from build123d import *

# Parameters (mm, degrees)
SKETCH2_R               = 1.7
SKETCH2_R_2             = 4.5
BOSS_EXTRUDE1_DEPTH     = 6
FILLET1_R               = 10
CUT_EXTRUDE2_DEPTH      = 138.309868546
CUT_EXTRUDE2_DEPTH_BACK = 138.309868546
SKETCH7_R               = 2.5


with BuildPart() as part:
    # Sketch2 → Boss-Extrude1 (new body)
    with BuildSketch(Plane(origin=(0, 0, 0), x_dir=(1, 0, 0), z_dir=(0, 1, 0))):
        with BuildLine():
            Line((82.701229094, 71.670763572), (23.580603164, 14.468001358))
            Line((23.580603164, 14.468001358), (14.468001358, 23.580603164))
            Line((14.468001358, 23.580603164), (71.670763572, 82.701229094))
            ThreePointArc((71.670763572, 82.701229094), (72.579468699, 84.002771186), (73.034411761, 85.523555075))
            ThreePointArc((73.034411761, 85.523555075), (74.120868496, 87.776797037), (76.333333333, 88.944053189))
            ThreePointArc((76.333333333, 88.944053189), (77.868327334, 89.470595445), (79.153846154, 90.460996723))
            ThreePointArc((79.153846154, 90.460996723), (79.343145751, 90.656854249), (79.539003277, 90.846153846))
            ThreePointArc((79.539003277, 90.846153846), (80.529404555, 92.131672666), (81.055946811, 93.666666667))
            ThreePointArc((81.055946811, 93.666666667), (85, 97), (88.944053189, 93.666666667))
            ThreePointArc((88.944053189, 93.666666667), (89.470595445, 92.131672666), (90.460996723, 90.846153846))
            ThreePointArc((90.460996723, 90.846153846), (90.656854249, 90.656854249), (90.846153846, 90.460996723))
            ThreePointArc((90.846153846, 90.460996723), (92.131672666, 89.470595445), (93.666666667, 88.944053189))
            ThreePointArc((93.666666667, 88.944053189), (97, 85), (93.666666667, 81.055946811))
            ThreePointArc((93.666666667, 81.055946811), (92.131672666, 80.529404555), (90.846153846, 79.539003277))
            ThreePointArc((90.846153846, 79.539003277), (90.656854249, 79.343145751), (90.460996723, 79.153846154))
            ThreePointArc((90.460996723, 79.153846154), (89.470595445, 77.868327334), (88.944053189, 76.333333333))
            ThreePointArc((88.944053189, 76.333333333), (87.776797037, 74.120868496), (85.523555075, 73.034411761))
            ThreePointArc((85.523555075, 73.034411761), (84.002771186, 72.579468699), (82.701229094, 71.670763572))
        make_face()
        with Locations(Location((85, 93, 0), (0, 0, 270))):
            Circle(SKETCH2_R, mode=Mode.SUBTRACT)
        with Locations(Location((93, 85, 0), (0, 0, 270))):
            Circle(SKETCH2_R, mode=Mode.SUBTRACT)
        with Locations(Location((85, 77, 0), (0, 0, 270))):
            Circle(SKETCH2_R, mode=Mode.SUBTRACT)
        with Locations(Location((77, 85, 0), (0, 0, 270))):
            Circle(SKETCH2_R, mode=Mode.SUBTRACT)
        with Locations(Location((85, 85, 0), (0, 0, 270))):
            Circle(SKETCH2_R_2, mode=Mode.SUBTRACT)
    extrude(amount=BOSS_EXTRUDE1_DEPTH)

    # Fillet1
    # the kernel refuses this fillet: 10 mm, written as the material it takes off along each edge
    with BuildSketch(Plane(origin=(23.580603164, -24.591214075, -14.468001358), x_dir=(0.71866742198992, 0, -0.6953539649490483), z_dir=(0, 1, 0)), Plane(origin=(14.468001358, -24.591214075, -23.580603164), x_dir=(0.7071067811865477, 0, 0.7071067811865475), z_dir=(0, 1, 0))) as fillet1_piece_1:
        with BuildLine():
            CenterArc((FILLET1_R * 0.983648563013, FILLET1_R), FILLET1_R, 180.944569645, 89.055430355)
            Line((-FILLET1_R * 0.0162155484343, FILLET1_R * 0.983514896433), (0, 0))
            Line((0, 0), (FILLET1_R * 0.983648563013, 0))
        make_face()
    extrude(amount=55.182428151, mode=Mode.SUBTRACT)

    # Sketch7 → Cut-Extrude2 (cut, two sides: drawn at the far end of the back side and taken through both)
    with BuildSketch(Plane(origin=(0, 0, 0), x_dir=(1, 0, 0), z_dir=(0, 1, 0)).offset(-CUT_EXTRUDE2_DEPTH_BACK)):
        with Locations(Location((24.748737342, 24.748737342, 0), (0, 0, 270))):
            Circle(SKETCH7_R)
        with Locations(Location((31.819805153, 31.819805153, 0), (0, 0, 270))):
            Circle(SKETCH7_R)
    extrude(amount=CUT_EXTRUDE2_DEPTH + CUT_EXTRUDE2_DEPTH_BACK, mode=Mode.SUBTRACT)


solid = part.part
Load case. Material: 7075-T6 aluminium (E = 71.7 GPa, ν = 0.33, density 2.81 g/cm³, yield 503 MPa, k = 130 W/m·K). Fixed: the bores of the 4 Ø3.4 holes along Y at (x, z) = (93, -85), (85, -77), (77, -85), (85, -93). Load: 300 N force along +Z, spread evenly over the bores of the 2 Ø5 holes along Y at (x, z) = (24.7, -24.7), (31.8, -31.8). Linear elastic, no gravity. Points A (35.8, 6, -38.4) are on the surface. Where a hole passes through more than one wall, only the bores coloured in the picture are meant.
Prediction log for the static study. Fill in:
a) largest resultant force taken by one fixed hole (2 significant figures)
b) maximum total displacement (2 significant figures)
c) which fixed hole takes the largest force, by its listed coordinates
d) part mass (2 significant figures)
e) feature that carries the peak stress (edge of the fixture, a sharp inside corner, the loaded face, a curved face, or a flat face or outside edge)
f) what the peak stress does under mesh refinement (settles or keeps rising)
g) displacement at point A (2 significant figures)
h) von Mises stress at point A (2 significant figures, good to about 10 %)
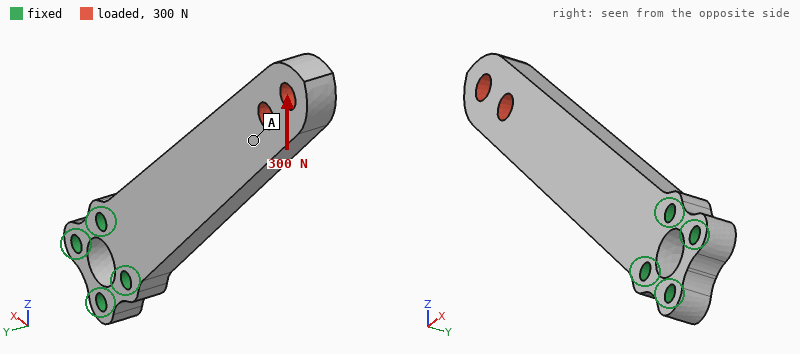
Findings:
1.4 kN
0.29 mm
(77, -85)
23 g
edge of the fixture
keeps rising
0.17 mm
8.2 MPa
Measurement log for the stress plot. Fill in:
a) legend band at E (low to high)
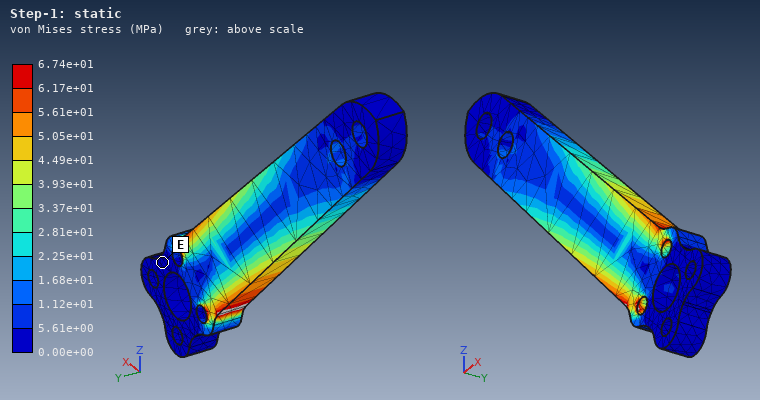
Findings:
0.00e+00 to 5.61e+00 MPa
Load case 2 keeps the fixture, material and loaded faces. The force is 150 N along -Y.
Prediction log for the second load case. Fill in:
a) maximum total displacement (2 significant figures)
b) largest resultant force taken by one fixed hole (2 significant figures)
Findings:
1.3 mm
93 N
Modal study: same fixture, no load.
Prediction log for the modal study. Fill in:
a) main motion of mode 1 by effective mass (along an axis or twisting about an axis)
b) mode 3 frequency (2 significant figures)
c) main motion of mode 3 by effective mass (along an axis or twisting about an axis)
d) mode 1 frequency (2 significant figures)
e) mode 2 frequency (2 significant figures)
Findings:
along Y
4400 Hz
along Y
770 Hz
2000 Hz
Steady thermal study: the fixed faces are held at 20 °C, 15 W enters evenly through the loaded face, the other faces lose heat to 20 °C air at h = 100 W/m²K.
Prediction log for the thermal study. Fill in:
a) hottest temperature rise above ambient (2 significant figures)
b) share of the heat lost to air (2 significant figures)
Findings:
58 K
59 %
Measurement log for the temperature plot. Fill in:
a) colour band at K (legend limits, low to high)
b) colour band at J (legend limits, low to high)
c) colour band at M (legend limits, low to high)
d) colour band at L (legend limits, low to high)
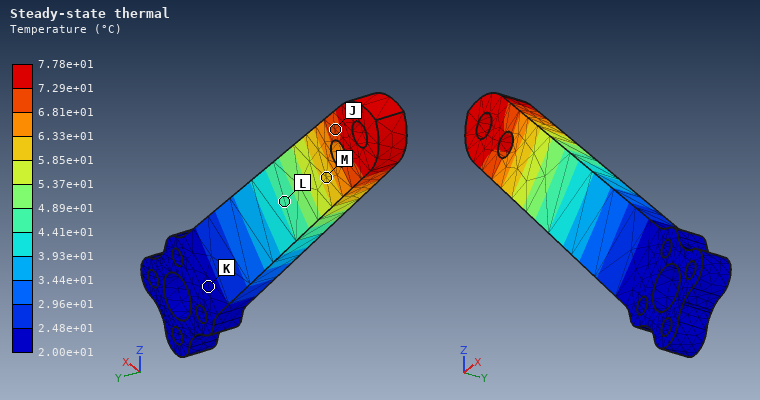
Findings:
2.00e+01 to 2.48e+01 °C
6.81e+01 to 7.29e+01 °C
5.85e+01 to 6.33e+01 °C
4.41e+01 to 4.89e+01 °C
